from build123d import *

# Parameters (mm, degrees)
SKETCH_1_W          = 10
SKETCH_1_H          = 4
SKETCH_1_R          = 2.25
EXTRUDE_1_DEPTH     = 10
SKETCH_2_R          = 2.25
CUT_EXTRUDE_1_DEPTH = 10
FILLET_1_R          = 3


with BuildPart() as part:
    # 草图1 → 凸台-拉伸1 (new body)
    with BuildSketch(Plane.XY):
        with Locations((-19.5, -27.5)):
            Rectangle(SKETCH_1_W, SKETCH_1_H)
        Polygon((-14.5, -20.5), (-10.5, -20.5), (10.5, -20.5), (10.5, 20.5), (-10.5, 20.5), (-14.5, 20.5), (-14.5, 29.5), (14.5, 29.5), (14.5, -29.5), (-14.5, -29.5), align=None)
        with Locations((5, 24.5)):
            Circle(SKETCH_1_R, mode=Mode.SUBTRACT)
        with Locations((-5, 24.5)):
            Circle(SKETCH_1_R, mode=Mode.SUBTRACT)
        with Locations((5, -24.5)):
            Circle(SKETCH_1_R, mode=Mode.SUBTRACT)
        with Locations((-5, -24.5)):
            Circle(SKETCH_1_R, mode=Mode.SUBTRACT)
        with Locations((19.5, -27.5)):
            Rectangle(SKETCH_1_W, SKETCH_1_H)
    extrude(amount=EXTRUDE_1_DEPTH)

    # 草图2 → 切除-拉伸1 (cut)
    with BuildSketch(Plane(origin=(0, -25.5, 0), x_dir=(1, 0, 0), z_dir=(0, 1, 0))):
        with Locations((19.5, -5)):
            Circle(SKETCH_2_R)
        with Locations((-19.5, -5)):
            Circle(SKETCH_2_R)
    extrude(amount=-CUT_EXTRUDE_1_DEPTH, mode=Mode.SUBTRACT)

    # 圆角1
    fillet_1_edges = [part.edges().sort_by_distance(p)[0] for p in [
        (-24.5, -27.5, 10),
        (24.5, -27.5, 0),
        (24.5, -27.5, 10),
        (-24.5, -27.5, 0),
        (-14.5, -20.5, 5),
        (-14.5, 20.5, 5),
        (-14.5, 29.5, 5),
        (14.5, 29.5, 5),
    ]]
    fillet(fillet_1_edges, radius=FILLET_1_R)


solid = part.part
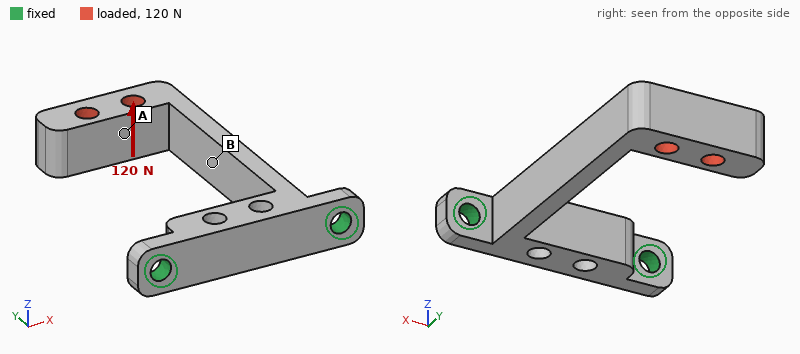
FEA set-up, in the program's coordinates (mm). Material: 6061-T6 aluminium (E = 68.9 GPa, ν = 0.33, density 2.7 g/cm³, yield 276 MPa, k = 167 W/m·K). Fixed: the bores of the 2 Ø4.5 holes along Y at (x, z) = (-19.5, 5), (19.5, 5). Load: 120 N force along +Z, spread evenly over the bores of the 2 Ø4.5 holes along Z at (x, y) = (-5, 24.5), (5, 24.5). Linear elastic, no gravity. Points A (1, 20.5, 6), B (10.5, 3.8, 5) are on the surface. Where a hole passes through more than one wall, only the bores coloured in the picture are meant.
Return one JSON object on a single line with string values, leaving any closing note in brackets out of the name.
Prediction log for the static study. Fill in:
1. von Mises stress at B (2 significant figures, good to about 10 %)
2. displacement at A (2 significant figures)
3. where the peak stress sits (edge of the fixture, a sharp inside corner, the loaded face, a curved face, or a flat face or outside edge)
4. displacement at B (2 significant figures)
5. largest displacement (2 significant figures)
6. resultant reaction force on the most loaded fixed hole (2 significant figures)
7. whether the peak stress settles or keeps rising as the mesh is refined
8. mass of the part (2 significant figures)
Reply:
{"von Mises stress at B": "68 MPa", "displacement at A": "0.54 mm", "where the peak stress sits": "edge of the fixture", "displacement at B": "0.22 mm", "largest displacement": "0.85 mm", "resultant reaction force on the most loaded fixed hole": "60 N", "whether the peak stress settles or keeps rising as the mesh is refined": "keeps rising", "mass of the part": "18 g"}
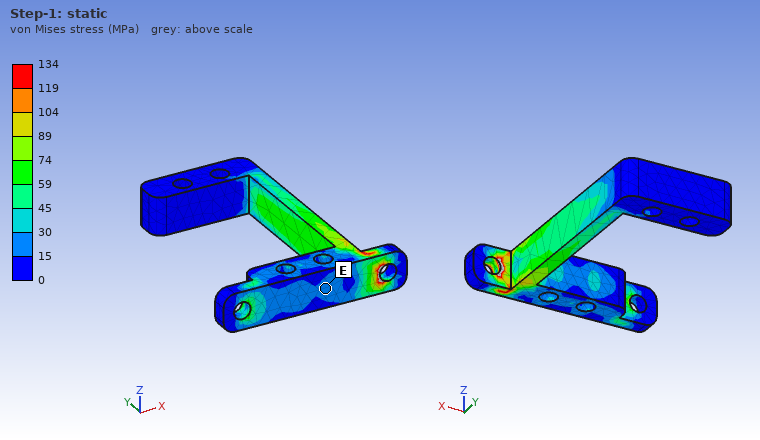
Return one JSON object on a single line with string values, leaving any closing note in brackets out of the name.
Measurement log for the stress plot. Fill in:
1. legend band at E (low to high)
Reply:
{"legend band at E": "15 to 30 MPa"}
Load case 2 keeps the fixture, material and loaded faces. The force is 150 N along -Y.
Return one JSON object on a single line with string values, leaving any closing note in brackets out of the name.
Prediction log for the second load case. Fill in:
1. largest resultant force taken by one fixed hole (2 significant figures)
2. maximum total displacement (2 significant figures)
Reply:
{"largest resultant force taken by one fixed hole": "130 N", "maximum total displacement": "0.91 mm"}
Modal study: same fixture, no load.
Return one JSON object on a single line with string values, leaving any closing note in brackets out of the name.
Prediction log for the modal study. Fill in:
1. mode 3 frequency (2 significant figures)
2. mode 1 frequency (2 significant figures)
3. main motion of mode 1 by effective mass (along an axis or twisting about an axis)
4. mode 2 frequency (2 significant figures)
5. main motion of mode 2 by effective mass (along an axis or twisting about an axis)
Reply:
{"mode 3 frequency": "2300 Hz", "mode 1 frequency": "550 Hz", "main motion of mode 1 by effective mass": "along X", "mode 2 frequency": "860 Hz", "main motion of mode 2 by effective mass": "along Z"}
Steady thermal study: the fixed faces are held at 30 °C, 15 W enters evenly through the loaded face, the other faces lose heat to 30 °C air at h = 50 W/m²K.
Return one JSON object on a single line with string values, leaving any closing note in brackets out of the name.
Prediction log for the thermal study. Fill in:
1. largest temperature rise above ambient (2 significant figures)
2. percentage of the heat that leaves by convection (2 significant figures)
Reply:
{"largest temperature rise above ambient": "82 K", "percentage of the heat that leaves by convection": "45 %"}
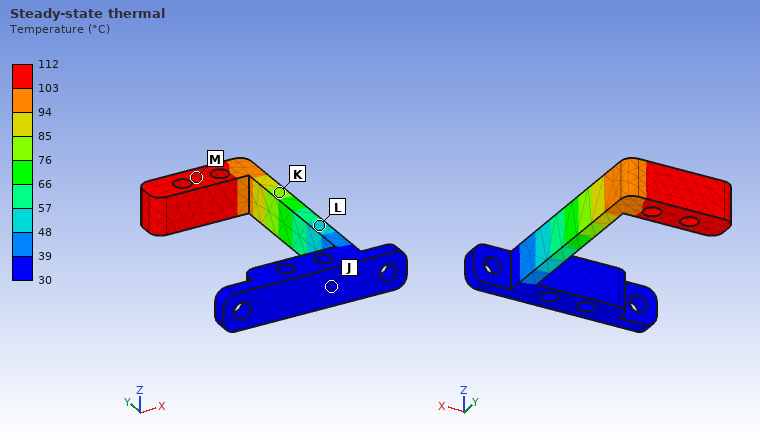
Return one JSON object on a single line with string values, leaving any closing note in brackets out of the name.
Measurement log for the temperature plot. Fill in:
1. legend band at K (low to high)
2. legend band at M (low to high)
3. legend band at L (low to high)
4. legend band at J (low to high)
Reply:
{"legend band at K": "76 to 85 °C", "legend band at M": "103 to 112 °C", "legend band at L": "48 to 57 °C", "legend band at J": "30 to 39 °C"}
